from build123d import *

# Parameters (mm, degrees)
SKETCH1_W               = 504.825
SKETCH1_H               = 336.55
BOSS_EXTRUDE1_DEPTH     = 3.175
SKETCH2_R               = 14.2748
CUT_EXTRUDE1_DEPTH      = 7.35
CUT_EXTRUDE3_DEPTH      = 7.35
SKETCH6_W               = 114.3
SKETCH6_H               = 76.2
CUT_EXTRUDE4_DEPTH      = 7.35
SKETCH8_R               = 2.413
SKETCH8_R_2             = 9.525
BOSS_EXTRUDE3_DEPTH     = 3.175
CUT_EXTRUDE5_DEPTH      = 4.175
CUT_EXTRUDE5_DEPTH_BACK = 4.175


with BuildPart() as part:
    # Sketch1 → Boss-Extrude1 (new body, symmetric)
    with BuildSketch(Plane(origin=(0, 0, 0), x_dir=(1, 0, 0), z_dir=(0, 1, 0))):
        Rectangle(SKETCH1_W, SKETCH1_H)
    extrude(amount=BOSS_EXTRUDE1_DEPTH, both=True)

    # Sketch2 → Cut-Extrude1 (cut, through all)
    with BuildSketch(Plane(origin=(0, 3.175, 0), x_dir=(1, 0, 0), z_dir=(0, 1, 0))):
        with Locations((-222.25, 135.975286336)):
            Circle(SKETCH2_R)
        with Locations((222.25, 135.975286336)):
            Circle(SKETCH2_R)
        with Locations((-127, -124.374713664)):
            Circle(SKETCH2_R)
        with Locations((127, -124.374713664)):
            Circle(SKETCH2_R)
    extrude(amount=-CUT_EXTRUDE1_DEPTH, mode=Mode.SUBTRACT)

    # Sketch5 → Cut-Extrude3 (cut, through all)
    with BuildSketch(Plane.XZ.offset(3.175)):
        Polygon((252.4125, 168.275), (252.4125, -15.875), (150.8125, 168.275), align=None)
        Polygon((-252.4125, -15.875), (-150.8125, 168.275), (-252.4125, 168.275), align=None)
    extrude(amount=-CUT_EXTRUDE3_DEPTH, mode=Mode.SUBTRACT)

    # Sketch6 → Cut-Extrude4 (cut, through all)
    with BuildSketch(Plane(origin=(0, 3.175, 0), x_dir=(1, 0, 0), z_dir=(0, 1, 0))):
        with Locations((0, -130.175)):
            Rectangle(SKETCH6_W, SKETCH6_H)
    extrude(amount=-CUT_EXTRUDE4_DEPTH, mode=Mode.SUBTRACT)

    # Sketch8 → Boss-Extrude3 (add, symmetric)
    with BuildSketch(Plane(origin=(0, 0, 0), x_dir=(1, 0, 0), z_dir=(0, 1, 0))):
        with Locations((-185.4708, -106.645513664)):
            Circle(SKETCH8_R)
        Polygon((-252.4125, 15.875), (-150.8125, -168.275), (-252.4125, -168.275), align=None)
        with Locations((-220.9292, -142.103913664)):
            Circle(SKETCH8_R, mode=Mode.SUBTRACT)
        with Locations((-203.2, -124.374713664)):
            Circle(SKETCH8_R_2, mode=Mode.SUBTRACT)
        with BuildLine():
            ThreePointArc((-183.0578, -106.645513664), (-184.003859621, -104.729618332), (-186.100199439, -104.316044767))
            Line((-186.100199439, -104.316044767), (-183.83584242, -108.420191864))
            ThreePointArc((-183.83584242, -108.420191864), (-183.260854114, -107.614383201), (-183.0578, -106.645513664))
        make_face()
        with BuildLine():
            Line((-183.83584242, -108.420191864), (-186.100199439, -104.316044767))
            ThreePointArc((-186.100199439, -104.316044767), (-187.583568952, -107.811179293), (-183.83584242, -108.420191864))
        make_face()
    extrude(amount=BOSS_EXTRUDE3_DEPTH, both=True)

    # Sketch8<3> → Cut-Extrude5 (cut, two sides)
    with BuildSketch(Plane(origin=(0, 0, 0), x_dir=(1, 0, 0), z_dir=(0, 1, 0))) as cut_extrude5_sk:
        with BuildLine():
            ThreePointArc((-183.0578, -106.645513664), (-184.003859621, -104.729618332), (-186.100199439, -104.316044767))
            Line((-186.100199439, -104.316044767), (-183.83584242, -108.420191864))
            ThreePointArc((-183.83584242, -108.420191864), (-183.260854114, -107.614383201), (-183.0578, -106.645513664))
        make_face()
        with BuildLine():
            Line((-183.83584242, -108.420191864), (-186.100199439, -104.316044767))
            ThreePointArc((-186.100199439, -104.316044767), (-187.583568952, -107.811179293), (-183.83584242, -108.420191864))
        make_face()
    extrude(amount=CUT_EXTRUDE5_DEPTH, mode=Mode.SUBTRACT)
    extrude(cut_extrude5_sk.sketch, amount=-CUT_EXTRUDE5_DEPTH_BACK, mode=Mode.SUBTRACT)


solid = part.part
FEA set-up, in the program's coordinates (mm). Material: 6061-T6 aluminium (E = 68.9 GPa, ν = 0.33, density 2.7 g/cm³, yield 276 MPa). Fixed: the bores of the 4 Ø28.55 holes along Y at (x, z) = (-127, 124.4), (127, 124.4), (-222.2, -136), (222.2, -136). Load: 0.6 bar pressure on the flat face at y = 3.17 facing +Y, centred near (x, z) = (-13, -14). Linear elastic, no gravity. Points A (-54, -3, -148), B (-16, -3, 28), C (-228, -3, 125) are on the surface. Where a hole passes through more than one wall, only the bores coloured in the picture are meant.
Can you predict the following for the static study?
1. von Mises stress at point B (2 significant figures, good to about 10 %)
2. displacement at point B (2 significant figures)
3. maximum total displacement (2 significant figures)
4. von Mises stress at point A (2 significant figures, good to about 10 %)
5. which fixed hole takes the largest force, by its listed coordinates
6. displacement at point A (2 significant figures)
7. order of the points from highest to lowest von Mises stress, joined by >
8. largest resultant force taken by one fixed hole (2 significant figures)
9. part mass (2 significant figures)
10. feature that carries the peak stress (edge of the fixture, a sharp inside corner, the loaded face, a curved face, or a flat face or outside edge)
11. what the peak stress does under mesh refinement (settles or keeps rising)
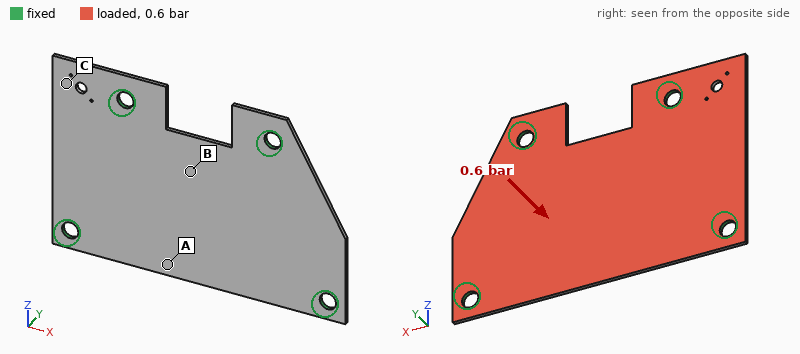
32 MPa
1.6 mm
3.7 mm
56 MPa
(-127, 124.4)
3.1 mm
A > B > C
2.5 kN
2.6 kg
edge of the fixture
keeps rising
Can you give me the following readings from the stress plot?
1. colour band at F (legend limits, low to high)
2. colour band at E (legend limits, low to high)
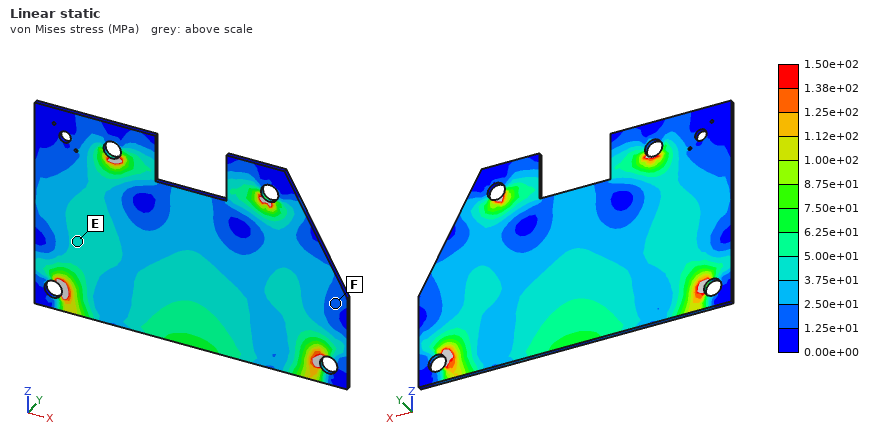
1.25e+01 to 2.50e+01 MPa
3.75e+01 to 5.00e+01 MPa
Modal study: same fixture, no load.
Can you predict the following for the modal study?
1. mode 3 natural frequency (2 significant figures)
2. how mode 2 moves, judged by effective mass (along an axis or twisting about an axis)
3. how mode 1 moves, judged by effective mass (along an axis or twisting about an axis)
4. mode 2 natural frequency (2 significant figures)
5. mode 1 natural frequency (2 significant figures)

430 Hz
along Y
along Y
380 Hz
200 Hz
